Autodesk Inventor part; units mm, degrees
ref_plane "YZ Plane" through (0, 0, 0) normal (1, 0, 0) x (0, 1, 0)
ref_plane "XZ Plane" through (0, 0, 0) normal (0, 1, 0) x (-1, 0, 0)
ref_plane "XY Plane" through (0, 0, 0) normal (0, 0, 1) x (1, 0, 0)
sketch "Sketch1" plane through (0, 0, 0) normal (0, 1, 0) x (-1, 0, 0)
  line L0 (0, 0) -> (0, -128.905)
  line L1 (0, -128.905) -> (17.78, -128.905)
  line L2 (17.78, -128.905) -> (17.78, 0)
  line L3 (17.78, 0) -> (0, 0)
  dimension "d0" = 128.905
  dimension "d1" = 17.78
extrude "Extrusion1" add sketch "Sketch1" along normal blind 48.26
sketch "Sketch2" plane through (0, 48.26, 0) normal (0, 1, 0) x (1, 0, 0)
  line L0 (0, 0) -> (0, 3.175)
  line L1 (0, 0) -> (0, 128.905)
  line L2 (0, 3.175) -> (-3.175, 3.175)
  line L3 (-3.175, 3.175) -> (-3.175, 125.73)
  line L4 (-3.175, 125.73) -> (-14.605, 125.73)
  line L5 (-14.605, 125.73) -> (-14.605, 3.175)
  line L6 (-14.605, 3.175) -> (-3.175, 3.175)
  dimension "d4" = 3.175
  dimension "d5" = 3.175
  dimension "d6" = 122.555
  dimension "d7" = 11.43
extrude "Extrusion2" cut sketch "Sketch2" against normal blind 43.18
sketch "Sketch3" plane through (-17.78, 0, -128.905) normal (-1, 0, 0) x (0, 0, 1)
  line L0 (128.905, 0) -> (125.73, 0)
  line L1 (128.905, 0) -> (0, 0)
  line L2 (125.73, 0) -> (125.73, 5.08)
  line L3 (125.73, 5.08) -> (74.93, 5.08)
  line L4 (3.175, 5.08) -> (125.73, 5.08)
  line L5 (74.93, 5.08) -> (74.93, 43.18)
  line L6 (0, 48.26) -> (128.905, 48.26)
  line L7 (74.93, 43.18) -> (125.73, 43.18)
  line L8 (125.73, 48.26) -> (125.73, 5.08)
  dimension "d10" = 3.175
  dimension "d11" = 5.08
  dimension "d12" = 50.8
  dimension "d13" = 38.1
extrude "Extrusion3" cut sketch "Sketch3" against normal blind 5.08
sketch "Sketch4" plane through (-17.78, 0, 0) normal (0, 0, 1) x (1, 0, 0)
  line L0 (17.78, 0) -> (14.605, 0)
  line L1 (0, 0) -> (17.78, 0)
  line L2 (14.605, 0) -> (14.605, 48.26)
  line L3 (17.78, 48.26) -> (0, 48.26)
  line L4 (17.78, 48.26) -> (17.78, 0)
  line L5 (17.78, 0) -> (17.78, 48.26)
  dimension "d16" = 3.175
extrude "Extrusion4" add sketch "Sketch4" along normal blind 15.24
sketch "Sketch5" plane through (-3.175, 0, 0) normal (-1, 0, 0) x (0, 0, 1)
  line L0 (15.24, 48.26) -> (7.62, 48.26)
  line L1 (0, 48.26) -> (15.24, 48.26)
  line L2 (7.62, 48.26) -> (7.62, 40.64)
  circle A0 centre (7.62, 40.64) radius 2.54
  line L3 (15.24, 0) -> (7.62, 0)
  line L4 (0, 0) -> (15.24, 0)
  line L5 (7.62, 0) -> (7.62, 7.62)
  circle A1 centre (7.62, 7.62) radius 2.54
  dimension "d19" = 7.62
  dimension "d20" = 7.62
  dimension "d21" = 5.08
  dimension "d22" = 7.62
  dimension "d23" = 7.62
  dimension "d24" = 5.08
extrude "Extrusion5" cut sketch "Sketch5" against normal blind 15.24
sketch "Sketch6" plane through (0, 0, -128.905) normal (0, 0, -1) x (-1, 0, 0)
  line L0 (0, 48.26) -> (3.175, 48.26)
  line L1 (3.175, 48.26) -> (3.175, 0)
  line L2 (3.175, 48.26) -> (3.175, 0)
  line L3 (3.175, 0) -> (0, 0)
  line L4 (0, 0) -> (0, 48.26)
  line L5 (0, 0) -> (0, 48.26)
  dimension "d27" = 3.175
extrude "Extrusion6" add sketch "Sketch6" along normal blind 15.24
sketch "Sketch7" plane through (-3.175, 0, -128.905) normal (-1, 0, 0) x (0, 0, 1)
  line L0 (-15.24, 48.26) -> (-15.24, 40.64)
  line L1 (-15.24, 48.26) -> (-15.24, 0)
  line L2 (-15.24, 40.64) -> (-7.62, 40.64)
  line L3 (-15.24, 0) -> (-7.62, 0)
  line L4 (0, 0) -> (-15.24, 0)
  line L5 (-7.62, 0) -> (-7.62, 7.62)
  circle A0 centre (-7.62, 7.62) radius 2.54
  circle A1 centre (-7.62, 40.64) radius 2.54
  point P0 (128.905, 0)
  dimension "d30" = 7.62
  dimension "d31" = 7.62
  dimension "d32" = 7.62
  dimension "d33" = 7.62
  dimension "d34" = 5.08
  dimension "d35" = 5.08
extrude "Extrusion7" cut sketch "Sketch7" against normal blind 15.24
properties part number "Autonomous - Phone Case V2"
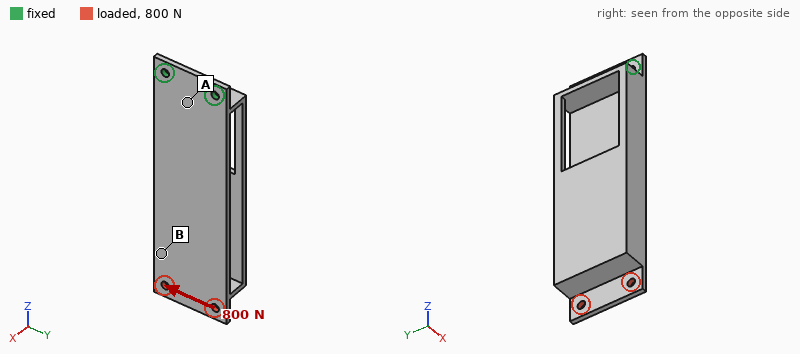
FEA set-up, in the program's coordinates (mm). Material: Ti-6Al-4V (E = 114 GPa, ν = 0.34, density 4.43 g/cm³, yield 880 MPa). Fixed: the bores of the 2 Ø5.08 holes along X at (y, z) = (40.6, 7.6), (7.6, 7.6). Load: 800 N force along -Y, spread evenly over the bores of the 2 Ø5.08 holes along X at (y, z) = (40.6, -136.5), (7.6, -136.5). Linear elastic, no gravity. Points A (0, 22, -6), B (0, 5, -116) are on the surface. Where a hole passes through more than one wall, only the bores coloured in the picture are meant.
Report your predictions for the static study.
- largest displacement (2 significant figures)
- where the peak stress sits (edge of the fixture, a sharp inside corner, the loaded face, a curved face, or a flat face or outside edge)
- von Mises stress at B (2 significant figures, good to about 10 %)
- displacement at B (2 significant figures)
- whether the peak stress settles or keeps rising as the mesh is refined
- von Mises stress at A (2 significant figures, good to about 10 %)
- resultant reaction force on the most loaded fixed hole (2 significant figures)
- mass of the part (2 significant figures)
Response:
0.27 mm
edge of the fixture
12 MPa
0.18 mm
keeps rising
27 MPa
3.3 kN
210 g
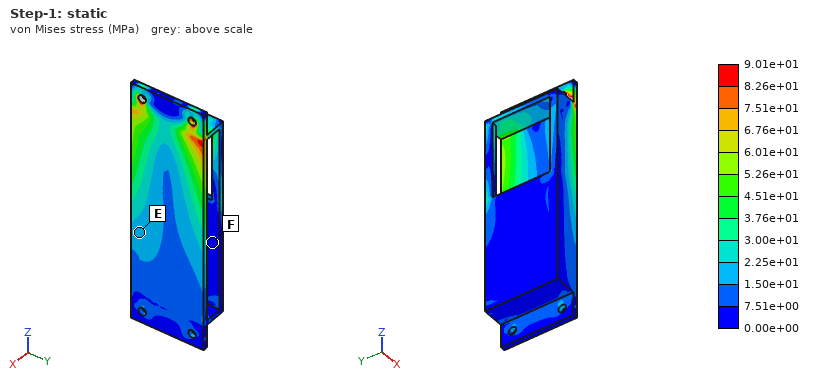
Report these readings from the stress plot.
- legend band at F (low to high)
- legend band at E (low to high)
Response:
0.00e+00 to 7.51e+00 MPa
1.50e+01 to 2.25e+01 MPa
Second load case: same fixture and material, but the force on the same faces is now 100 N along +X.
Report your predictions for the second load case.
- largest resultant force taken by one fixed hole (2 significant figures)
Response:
150 N
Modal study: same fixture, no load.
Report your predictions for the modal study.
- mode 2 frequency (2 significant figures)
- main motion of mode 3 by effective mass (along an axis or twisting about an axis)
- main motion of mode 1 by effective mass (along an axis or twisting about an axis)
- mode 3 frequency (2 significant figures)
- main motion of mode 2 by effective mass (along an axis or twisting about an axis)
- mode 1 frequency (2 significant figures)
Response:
740 Hz
along Y
along X
1200 Hz
along Y
140 Hz
